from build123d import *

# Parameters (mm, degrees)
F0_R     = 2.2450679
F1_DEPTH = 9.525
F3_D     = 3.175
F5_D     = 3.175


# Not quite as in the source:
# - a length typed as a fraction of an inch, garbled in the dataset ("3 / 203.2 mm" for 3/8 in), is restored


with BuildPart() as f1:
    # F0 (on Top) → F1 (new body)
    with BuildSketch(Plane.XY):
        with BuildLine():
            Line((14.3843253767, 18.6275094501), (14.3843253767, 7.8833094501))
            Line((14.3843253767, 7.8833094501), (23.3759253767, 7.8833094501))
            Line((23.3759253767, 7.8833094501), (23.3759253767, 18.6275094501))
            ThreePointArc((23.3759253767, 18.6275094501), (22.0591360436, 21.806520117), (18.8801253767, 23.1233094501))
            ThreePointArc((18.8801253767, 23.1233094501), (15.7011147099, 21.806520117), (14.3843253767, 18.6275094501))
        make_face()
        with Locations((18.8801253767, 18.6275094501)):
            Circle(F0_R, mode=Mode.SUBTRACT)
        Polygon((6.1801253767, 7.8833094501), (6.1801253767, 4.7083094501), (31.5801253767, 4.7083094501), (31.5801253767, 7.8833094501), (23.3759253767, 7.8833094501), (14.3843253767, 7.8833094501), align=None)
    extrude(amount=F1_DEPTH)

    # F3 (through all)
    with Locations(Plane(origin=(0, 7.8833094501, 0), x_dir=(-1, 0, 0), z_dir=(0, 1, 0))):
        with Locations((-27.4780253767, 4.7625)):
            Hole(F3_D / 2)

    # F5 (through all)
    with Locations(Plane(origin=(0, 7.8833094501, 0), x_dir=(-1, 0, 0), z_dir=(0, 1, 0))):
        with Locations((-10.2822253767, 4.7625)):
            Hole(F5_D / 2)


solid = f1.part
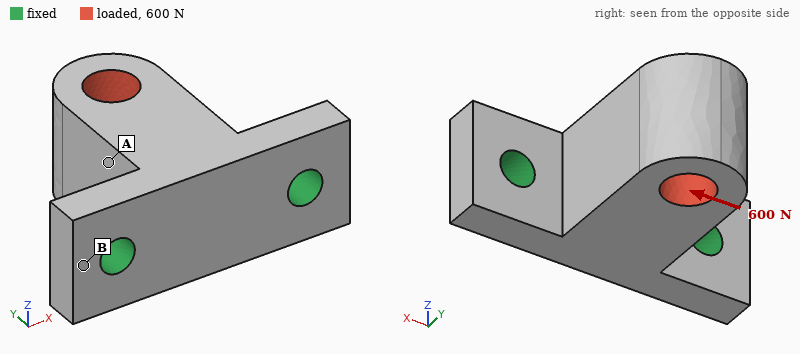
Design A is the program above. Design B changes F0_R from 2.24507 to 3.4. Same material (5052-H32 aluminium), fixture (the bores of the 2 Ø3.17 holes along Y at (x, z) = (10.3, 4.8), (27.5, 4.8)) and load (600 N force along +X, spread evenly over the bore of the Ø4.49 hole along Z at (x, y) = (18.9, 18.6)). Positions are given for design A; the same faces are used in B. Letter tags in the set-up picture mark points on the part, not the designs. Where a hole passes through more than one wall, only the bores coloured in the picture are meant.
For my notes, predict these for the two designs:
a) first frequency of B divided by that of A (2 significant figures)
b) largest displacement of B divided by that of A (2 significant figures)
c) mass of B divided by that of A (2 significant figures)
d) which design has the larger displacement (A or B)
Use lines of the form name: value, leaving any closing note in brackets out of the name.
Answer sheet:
first frequency of B divided by that of A: 1.2
largest displacement of B divided by that of A: 1.6
mass of B divided by that of A: 0.89
which design has the larger displacement: B
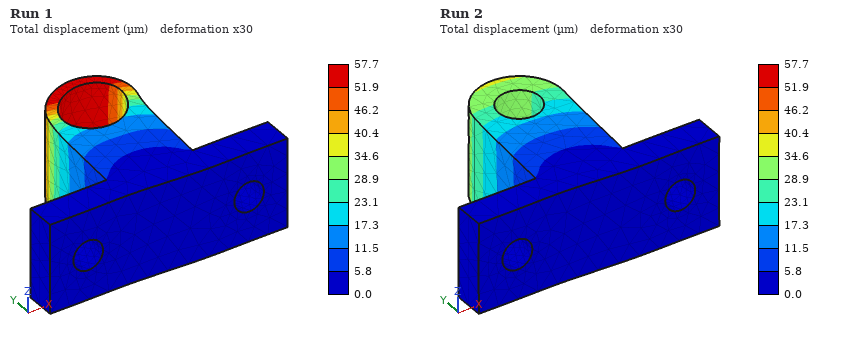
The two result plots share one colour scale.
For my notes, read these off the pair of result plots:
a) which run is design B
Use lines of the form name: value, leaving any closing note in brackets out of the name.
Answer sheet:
which run is design B: Run 1
